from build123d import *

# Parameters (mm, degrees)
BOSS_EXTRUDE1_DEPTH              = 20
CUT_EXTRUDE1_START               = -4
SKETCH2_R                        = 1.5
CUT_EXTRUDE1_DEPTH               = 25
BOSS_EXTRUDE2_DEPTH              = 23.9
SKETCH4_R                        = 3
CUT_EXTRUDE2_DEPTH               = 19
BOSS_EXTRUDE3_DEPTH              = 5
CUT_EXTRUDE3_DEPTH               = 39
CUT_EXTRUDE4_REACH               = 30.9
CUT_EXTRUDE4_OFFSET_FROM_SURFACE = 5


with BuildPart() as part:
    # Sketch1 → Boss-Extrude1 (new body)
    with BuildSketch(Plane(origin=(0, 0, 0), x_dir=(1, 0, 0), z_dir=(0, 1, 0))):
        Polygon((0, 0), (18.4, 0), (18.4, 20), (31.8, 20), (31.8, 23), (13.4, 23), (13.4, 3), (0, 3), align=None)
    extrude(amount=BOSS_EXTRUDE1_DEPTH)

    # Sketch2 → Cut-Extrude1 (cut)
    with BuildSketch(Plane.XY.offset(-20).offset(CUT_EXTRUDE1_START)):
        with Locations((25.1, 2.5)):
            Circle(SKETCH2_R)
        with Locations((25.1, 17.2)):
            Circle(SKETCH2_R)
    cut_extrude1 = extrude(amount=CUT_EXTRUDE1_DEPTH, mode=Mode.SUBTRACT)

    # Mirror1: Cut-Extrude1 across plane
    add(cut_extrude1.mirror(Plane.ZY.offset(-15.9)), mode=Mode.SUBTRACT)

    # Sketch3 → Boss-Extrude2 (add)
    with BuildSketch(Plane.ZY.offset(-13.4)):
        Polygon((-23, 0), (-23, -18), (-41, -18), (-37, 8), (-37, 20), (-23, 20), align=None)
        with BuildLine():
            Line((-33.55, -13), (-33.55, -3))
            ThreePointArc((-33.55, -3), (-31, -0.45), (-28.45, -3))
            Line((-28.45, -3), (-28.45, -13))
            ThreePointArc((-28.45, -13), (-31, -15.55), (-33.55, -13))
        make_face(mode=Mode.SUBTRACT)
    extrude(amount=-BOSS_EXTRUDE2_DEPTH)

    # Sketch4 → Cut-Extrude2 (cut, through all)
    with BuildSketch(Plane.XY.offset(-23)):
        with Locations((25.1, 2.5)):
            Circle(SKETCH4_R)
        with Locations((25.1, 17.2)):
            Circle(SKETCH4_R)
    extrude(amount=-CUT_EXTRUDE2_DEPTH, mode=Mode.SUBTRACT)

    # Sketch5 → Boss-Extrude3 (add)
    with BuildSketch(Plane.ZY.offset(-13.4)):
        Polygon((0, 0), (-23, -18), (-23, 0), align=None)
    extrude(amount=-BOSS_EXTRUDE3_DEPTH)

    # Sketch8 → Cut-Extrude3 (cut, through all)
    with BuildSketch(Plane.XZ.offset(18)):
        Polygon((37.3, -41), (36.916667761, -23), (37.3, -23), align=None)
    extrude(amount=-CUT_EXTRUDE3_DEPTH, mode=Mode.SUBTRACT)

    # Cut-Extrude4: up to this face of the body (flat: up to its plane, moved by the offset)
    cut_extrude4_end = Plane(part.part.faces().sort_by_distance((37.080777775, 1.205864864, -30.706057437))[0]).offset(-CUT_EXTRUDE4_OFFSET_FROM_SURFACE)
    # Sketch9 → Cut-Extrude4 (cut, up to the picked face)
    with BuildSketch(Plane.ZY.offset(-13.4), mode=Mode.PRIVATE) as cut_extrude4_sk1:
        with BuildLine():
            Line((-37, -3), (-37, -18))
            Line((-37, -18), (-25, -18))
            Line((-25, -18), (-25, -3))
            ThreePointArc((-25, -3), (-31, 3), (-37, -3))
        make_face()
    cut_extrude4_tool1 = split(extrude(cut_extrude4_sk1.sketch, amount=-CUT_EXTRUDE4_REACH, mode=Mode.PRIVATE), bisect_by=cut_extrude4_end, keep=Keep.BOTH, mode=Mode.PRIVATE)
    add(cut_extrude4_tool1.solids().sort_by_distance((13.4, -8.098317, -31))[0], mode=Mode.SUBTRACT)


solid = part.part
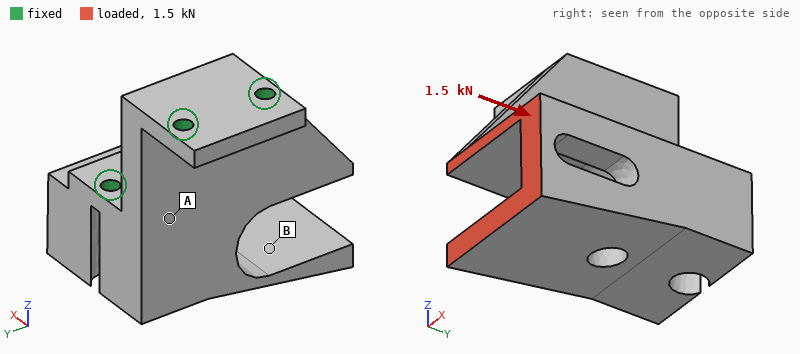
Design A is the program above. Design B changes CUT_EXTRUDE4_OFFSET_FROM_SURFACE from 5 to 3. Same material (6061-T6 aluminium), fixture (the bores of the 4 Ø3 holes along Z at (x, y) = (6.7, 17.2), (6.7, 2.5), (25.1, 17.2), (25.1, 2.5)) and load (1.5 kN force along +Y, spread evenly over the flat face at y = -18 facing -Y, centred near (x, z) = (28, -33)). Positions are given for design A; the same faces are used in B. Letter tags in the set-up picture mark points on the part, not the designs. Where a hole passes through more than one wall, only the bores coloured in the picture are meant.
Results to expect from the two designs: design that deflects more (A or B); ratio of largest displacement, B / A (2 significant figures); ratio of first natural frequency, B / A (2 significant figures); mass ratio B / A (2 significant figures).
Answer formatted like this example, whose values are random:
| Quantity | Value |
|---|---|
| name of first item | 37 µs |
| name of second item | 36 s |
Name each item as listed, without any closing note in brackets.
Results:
| Quantity | Value |
|---|---|
| design that deflects more | B |
| ratio of largest displacement, B / A | 1.4 |
| ratio of first natural frequency, B / A | 0.92 |
| mass ratio B / A | 0.98 |
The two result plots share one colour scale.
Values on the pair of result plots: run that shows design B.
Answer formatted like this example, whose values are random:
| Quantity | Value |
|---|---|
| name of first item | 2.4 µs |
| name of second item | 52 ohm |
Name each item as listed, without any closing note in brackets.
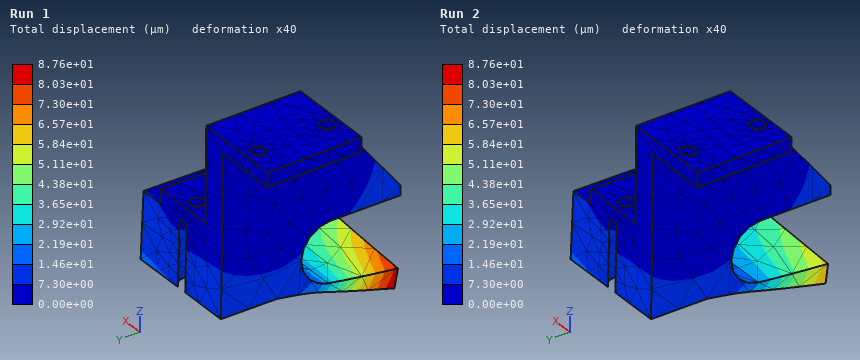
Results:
| Quantity | Value |
|---|---|
| run that shows design B | Run 1 |
